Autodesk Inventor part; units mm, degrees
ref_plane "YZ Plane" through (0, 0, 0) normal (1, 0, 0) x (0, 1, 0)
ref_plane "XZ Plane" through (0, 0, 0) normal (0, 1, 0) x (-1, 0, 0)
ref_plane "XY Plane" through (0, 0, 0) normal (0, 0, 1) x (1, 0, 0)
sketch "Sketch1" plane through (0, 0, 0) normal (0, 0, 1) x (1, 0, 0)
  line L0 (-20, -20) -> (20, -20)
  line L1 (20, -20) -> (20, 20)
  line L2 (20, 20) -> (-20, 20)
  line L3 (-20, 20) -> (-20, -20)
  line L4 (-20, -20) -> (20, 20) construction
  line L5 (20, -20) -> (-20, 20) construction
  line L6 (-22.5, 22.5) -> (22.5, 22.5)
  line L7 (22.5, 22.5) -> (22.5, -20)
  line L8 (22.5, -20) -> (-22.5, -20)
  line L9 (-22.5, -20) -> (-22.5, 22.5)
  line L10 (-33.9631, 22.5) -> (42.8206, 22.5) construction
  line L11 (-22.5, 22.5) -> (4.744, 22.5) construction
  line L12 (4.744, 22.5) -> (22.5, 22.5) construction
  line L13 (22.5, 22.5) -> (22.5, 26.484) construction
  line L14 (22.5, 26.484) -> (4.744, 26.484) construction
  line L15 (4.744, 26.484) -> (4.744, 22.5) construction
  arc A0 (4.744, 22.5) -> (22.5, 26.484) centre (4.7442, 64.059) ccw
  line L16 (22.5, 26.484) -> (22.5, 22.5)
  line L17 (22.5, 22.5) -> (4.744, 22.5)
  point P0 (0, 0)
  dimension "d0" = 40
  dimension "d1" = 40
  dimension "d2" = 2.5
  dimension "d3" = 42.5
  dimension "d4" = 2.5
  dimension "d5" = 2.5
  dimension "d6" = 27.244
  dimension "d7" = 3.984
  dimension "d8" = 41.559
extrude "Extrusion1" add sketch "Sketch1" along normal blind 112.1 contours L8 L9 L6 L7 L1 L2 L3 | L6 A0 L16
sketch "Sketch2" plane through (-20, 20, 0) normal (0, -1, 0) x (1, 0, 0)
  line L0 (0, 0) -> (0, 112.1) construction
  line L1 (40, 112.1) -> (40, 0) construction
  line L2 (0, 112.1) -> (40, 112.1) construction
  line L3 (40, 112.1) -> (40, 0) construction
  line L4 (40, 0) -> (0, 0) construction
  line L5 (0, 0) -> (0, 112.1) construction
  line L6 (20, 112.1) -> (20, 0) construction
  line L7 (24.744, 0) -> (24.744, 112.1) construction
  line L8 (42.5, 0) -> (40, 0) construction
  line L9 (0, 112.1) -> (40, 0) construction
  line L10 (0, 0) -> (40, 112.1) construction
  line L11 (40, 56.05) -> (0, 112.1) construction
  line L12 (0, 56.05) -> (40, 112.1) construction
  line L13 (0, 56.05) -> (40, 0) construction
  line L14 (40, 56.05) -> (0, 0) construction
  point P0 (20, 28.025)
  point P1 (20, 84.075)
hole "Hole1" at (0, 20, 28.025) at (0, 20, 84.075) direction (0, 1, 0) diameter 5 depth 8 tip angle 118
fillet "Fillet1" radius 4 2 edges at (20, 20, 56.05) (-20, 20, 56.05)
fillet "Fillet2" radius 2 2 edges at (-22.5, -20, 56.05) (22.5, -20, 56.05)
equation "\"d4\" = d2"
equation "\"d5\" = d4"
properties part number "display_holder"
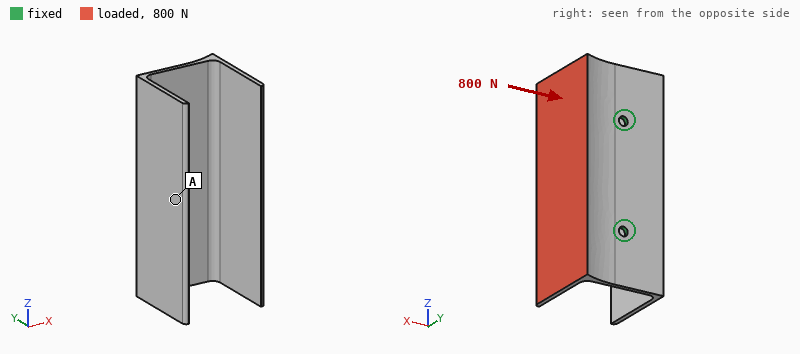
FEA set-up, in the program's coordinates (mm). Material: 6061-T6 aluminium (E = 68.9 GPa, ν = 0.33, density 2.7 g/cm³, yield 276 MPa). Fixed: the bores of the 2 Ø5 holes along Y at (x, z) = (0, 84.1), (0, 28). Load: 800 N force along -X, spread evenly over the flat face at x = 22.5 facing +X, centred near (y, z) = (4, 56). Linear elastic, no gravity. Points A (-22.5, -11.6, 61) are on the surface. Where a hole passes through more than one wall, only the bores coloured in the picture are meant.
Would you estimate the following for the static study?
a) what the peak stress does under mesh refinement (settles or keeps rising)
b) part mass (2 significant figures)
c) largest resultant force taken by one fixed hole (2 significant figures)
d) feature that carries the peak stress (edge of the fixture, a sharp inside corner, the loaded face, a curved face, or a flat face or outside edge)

keeps rising
100 g
400 N
edge of the fixture
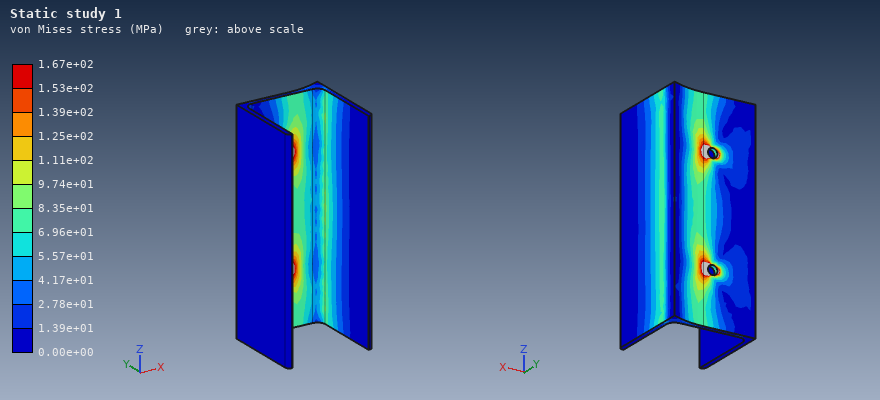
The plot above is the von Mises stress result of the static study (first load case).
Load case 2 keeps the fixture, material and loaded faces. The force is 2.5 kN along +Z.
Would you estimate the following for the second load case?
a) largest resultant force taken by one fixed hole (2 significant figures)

1.7 kN
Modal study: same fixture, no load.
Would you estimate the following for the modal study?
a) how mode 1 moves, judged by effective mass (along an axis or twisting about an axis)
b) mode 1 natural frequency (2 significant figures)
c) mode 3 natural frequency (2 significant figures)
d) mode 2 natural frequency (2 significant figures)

along X
630 Hz
1000 Hz
790 Hz
